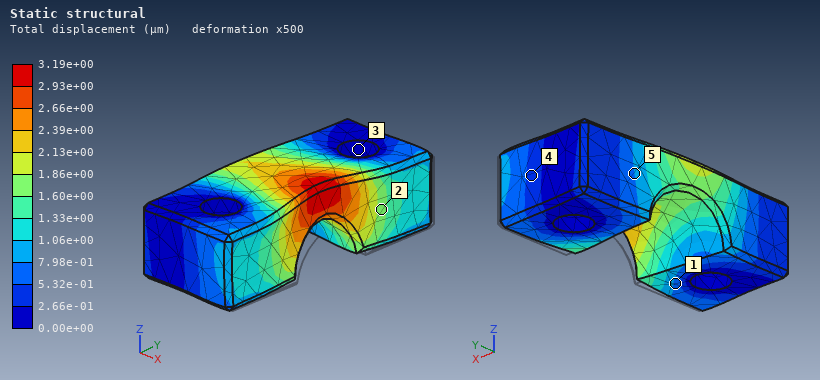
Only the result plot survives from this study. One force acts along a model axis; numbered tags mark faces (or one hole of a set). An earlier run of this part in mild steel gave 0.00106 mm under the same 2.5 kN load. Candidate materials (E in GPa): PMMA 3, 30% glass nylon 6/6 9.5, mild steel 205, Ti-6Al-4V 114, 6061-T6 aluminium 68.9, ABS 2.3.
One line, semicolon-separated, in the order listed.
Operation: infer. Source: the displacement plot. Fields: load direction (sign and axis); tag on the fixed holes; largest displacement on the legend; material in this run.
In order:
-X; 3; 3.19e+00 µm; 6061-T6 aluminium
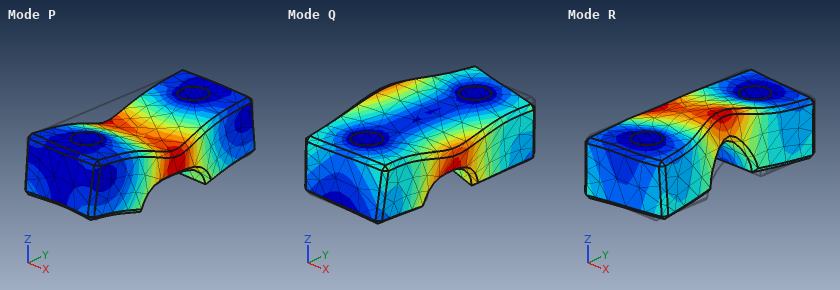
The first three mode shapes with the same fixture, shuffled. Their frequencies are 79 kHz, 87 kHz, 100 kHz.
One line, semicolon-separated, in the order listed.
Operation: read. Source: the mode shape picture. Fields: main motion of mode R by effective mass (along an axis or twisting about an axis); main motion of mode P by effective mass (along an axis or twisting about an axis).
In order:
along X; along Z
